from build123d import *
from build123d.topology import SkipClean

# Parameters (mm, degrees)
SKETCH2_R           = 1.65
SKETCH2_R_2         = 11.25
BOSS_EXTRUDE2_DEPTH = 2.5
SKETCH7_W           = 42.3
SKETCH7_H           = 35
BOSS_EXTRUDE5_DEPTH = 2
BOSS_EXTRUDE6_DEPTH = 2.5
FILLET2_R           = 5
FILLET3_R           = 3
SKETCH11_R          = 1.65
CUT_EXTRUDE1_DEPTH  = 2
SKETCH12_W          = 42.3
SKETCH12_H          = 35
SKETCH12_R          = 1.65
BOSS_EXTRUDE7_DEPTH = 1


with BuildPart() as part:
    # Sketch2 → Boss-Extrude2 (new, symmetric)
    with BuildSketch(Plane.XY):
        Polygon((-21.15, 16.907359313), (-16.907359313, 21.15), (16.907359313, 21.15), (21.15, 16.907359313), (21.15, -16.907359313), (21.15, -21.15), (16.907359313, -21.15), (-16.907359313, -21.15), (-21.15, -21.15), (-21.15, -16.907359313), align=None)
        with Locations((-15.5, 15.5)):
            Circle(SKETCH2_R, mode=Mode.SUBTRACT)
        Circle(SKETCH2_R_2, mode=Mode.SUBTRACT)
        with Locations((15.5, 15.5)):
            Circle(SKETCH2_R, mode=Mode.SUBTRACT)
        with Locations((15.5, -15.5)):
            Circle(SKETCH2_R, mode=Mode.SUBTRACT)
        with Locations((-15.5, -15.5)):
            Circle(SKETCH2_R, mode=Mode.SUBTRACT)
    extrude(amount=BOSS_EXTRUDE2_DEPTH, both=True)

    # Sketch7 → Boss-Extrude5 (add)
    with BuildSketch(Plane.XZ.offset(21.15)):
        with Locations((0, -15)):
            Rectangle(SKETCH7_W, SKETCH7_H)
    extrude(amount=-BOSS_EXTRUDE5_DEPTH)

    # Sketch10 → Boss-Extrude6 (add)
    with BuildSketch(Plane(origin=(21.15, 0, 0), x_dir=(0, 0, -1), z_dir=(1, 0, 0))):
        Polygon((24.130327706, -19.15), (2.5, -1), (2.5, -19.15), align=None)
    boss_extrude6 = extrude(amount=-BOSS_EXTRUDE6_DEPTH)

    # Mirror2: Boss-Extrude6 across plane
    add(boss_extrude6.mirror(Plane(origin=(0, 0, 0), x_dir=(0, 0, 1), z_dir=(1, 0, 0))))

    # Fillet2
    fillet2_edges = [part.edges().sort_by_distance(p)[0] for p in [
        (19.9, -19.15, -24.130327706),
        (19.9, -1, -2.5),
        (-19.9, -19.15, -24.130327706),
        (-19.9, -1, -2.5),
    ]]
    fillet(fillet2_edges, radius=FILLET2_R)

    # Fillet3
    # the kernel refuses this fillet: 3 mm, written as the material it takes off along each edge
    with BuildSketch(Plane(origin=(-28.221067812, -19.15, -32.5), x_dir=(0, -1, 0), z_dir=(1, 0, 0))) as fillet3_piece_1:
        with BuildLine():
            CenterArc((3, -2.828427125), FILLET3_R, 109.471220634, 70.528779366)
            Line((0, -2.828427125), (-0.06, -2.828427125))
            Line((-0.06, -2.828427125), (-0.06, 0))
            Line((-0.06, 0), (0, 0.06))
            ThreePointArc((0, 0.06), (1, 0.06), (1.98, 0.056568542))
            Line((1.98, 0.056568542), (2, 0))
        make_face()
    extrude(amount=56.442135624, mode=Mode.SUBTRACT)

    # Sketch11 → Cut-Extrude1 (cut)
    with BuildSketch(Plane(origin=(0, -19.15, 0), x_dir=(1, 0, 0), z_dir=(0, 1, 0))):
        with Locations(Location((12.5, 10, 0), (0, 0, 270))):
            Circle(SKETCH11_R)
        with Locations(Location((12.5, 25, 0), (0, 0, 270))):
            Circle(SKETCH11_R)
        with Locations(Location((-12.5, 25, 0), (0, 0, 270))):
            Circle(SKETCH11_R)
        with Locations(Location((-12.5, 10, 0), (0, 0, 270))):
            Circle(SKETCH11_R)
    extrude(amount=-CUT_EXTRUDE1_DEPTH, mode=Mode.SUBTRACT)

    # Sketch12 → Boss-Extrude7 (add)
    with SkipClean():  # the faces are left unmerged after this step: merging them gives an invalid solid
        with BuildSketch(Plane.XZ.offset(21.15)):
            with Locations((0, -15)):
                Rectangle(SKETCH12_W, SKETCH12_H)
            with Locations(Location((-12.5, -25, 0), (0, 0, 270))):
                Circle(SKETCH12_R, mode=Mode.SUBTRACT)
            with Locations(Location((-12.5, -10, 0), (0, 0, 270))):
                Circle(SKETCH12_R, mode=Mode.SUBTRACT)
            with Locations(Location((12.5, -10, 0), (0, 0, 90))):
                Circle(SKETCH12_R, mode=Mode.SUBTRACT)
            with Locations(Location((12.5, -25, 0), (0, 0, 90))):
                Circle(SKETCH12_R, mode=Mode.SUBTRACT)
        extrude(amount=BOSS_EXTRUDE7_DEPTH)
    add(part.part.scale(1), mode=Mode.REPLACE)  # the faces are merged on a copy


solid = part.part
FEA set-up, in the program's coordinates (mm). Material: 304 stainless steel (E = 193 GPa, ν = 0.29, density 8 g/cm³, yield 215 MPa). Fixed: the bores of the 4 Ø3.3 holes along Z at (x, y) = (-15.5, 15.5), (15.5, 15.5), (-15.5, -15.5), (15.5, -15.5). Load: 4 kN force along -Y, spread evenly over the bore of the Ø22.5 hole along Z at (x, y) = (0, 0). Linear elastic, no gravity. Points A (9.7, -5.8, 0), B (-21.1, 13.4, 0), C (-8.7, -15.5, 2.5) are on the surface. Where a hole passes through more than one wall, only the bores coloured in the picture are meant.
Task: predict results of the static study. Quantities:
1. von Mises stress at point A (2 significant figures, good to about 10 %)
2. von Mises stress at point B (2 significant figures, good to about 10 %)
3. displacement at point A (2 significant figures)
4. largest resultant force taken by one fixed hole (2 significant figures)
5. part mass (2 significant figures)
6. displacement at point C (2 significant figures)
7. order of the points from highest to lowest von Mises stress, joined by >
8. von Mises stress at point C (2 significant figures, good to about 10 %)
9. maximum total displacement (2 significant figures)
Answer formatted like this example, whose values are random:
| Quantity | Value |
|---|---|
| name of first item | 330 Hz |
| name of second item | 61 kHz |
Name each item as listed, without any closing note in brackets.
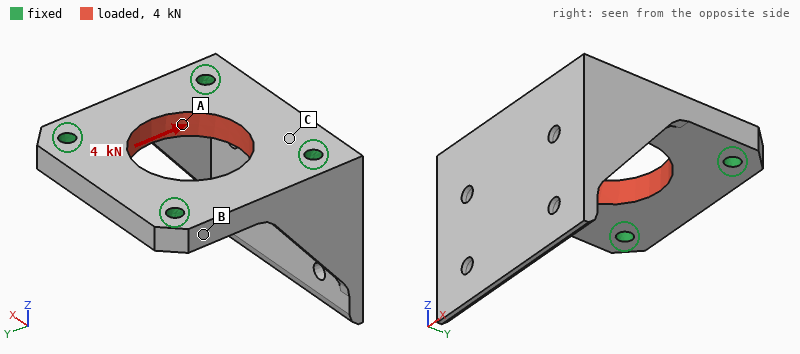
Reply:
| Quantity | Value |
|---|---|
| von Mises stress at point A | 24 MPa |
| von Mises stress at point B | 5.6 MPa |
| displacement at point A | 1.2 µm |
| largest resultant force taken by one fixed hole | 1.0 kN |
| part mass | 92 g |
| displacement at point C | 1.1 µm |
| order of the points from highest to lowest von Mises stress, joined by > | A > C > B |
| von Mises stress at point C | 14 MPa |
| maximum total displacement | 2.7 µm |
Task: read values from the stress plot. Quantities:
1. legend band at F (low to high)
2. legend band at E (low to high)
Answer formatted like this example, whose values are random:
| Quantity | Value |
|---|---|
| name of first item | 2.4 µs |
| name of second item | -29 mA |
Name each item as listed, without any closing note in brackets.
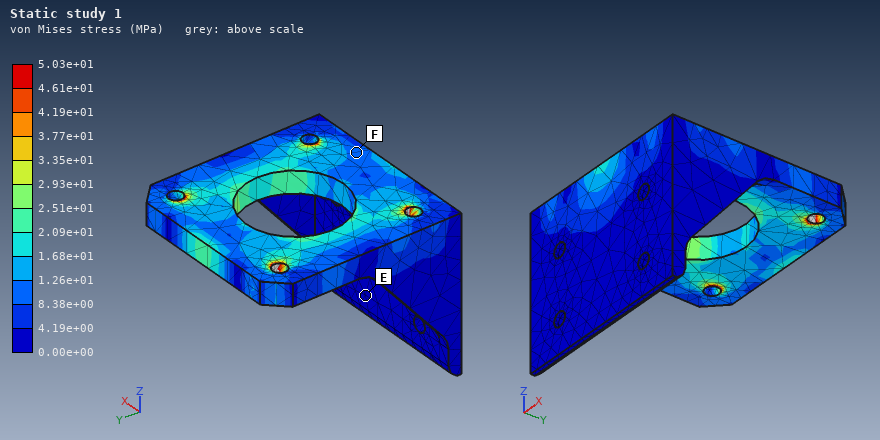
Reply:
| Quantity | Value |
|---|---|
| legend band at F | 8.38e+00 to 1.26e+01 MPa |
| legend band at E | 0.00e+00 to 4.19e+00 MPa |
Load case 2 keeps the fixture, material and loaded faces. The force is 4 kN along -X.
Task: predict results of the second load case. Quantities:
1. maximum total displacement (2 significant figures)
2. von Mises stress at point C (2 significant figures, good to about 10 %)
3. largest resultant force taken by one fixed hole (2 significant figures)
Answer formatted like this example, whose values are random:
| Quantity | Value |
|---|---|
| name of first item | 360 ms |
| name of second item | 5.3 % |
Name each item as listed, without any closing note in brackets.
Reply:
| Quantity | Value |
|---|---|
| maximum total displacement | 2.6 µm |
| von Mises stress at point C | 14 MPa |
| largest resultant force taken by one fixed hole | 1.0 kN |
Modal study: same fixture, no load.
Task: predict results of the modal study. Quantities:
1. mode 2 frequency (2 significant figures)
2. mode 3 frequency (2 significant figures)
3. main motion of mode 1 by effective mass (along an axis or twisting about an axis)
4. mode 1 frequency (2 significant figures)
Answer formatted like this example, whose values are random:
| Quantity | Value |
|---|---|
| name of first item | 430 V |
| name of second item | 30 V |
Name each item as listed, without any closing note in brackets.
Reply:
| Quantity | Value |
|---|---|
| mode 2 frequency | 8900 Hz |
| mode 3 frequency | 14 kHz |
| main motion of mode 1 by effective mass | along Y |
| mode 1 frequency | 4700 Hz |
